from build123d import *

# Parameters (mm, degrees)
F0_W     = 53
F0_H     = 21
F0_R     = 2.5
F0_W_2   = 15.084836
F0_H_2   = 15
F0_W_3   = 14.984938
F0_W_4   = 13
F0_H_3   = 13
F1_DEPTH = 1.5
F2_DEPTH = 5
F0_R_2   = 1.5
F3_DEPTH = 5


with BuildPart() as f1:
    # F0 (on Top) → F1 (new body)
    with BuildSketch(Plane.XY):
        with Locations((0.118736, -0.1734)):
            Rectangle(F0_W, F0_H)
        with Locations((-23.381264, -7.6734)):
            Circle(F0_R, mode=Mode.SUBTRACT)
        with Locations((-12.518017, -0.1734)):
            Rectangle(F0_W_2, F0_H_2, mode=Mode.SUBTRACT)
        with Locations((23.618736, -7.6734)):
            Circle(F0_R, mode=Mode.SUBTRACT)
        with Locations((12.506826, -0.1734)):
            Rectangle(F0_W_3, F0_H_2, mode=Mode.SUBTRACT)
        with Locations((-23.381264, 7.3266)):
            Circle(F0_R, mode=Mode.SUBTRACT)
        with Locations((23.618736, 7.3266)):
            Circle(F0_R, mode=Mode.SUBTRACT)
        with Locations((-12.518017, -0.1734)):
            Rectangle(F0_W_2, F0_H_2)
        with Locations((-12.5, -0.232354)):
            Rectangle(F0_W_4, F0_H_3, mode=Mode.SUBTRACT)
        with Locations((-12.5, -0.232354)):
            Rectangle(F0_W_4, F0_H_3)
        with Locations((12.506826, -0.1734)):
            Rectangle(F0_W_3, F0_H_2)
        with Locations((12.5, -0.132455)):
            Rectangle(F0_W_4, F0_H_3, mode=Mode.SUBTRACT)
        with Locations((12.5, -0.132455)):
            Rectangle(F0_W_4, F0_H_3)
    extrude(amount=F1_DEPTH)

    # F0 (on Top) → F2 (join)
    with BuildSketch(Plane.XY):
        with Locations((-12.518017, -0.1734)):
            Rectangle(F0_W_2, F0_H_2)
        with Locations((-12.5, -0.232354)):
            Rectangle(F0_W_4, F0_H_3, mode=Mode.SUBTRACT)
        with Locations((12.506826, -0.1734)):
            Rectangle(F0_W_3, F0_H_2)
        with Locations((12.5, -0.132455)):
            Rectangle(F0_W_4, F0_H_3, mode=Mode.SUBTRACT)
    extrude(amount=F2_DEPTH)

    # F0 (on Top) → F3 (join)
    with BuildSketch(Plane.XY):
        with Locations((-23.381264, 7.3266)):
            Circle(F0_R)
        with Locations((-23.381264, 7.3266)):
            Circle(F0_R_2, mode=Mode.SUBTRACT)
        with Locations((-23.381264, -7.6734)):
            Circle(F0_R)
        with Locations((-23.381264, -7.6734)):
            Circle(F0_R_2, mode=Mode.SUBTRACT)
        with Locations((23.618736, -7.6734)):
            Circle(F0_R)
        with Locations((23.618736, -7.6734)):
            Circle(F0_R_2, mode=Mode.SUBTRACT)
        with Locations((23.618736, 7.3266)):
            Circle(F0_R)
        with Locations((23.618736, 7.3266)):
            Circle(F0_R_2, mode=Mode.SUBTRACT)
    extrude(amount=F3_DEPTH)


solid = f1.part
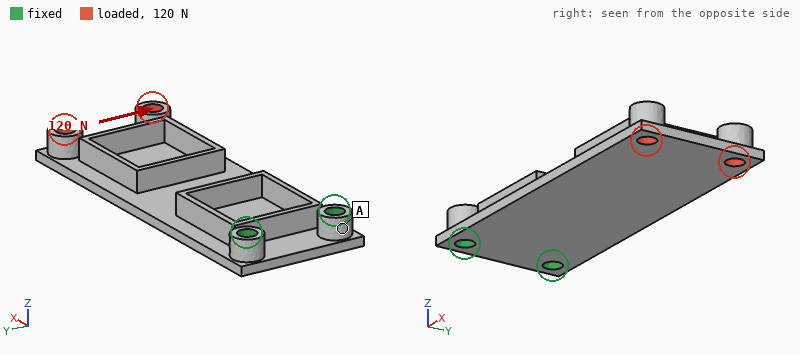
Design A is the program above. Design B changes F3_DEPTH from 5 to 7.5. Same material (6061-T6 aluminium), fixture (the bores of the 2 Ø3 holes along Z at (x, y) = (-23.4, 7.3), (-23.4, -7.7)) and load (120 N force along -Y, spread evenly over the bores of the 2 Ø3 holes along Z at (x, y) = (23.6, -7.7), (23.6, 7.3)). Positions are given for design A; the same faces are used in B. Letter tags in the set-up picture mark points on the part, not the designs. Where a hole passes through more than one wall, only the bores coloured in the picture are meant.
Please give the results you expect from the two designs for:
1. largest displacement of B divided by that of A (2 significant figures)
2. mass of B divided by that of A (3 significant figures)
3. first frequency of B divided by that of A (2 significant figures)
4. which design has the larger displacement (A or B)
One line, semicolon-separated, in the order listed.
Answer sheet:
1.7; 1.06; 0.95; B
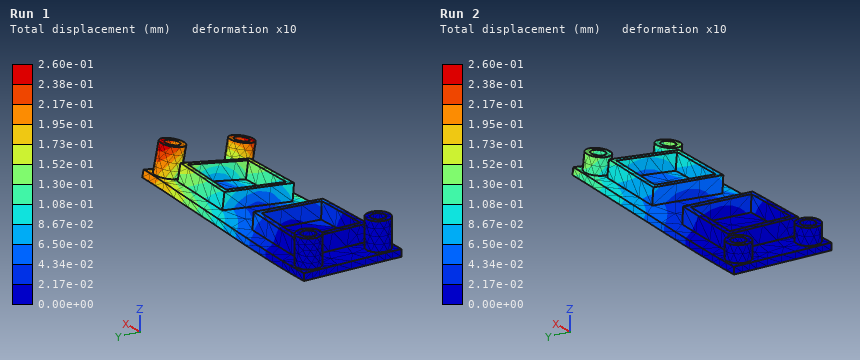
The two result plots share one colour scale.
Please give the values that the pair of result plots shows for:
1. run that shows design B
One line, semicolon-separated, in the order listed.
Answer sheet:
Run 1
